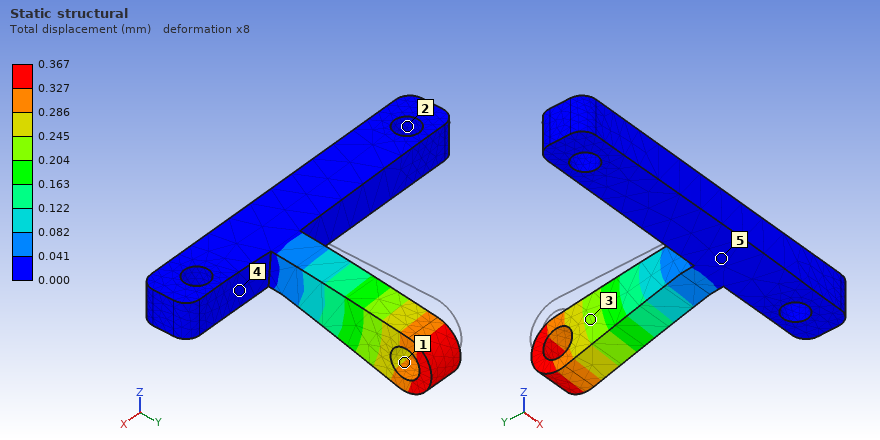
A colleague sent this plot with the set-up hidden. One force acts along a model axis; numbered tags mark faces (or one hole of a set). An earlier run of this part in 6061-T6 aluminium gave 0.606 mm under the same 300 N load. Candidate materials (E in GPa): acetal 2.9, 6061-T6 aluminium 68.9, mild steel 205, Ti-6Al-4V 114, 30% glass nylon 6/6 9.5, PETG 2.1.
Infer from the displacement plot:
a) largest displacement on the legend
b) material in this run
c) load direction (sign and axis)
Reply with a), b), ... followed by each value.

a) 0.367 mm
b) Ti-6Al-4V
c) -Z
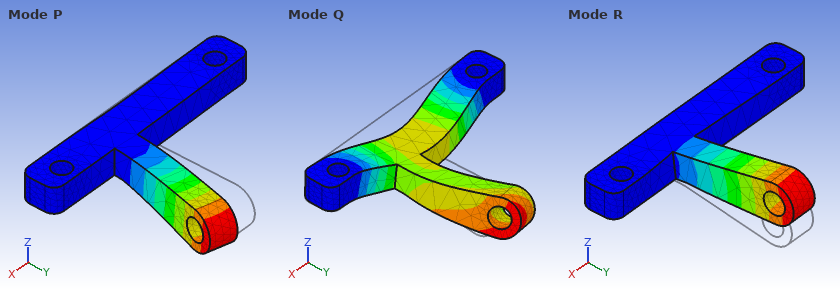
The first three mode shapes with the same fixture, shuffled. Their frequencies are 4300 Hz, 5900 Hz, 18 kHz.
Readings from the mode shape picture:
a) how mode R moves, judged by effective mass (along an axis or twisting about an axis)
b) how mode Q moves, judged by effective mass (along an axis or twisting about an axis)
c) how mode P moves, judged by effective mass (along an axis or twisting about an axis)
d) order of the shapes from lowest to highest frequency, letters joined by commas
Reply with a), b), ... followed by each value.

a) along Z
b) along Y
c) along X
d) R, P, Q
